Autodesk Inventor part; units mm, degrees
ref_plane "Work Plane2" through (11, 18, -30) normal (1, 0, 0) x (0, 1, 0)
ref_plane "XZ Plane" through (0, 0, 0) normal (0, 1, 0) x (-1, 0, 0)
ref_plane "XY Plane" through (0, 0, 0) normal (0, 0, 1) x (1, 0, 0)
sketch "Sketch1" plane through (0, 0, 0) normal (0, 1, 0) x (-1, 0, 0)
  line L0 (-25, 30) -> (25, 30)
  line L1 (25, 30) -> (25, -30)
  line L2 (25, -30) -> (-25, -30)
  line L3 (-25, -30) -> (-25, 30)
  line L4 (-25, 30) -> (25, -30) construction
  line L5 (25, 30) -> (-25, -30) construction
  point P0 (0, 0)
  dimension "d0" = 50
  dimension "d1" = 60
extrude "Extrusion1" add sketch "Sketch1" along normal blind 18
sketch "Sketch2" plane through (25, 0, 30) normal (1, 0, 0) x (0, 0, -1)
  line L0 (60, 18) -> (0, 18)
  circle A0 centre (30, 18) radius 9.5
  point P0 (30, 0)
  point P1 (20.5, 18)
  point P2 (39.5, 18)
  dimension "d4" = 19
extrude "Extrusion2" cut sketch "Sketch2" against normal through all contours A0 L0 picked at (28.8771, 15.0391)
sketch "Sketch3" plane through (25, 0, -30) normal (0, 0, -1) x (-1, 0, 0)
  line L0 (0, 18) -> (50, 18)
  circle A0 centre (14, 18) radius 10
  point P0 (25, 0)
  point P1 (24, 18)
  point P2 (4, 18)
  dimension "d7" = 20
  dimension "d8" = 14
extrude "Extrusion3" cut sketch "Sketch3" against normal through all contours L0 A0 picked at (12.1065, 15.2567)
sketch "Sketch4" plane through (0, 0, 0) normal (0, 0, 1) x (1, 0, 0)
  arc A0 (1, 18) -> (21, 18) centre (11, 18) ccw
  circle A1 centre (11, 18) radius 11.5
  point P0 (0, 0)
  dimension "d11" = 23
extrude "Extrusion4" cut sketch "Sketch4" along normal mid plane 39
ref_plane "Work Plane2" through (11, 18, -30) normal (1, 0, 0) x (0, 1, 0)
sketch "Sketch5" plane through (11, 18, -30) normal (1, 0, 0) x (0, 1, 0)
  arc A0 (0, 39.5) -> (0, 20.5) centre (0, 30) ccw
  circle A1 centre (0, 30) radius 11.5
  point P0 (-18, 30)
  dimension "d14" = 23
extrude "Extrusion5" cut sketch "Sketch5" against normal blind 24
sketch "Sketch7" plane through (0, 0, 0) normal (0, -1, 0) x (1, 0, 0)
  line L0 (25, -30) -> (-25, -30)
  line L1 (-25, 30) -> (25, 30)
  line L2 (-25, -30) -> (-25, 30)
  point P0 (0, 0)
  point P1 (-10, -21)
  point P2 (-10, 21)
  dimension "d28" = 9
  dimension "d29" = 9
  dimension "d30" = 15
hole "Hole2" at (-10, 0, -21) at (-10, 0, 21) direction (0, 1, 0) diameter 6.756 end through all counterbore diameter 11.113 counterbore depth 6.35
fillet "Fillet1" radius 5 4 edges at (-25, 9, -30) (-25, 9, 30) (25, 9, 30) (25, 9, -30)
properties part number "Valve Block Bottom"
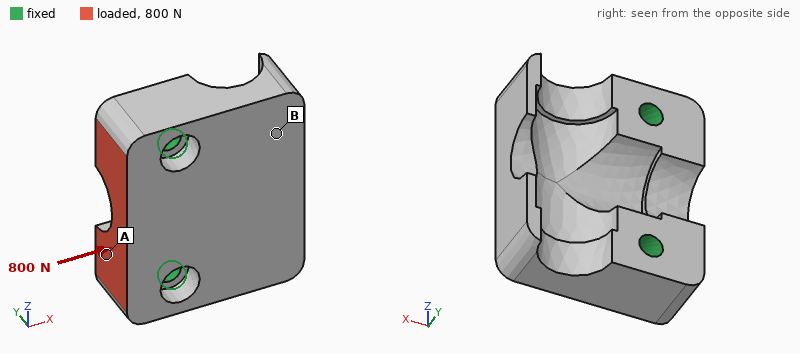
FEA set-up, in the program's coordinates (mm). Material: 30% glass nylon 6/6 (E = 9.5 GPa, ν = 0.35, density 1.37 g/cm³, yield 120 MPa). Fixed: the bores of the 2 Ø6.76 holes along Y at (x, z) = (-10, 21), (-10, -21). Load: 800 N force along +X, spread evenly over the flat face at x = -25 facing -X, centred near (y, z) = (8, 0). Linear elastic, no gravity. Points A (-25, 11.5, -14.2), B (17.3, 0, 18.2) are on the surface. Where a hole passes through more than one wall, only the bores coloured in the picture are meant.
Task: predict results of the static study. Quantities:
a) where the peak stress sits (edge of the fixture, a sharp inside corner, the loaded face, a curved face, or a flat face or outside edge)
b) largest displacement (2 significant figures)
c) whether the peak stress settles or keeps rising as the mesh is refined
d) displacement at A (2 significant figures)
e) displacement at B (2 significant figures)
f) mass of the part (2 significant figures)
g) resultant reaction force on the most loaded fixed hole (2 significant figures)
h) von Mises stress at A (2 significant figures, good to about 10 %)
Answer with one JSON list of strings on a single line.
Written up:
["edge of the fixture", "10 µm", "keeps rising", "4.8 µm", "7.9 µm", "48 g", "400 N", "1.2 MPa"]
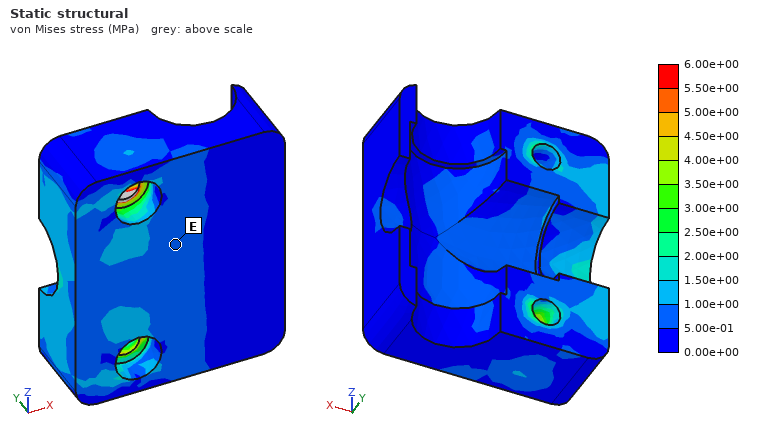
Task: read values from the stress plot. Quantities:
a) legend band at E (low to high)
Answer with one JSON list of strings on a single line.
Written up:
["5.00e-01 to 1.00e+00 MPa"]
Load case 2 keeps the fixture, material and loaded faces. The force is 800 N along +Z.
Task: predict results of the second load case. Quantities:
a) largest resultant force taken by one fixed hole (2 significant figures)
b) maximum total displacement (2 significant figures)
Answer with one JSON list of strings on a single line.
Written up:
["460 N", "10 µm"]
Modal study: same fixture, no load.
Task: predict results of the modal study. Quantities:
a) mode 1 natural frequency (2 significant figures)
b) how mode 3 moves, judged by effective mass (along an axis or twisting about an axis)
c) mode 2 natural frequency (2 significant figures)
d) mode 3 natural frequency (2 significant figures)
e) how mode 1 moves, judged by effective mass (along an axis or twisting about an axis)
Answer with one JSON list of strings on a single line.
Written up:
["3100 Hz", "along Z", "4500 Hz", "7700 Hz", "along Y"]
